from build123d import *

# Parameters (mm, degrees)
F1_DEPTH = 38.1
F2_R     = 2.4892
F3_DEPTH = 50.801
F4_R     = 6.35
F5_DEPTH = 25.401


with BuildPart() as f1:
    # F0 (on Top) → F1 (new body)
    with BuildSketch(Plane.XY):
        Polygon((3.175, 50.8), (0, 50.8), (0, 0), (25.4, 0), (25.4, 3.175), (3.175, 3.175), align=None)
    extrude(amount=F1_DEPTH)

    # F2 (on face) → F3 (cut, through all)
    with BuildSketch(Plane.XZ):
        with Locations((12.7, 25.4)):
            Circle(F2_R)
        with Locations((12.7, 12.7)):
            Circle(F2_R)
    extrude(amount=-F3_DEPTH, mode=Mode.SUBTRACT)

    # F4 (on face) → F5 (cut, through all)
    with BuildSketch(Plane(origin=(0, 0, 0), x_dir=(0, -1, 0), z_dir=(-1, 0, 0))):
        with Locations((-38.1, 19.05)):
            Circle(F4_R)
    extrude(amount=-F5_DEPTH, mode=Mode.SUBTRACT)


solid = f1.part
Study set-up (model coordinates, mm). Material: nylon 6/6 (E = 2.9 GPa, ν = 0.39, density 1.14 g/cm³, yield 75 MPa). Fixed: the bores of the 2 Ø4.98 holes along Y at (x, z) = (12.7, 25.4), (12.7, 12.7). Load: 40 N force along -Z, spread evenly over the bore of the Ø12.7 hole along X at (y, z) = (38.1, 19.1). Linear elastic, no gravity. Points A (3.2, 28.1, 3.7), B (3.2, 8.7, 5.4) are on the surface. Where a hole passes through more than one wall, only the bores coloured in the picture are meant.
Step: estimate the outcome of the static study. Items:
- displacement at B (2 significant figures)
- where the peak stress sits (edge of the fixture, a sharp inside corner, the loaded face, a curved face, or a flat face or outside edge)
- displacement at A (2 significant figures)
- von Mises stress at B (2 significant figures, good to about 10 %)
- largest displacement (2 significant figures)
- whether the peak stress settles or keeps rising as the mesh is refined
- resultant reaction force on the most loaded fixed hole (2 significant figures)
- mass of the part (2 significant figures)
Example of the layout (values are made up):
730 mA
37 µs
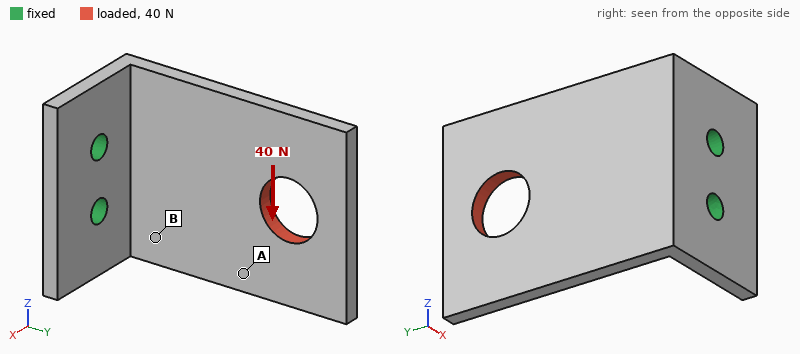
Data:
0.19 mm
edge of the fixture
0.41 mm
4.9 MPa
0.69 mm
keeps rising
81 N
9.5 g
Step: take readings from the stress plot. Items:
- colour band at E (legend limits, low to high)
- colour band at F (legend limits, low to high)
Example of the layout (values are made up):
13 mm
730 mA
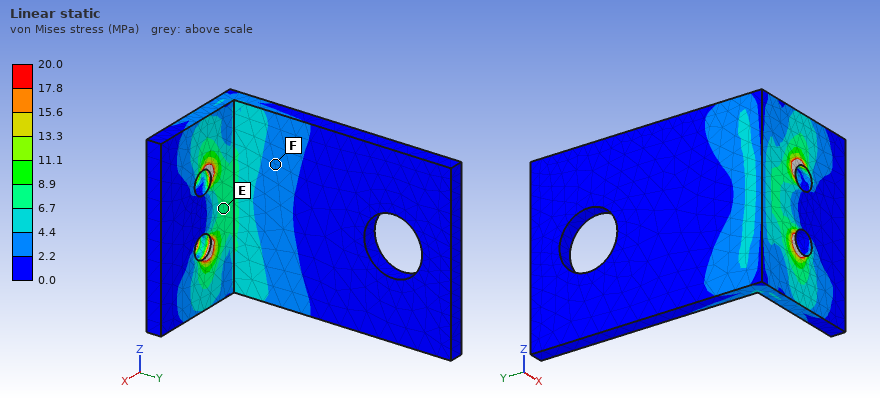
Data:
6.7 to 8.9 MPa
2.2 to 4.4 MPa
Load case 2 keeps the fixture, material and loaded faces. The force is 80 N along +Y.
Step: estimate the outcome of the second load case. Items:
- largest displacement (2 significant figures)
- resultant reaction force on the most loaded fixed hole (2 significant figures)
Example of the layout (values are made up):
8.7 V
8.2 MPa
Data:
0.68 mm
40 N
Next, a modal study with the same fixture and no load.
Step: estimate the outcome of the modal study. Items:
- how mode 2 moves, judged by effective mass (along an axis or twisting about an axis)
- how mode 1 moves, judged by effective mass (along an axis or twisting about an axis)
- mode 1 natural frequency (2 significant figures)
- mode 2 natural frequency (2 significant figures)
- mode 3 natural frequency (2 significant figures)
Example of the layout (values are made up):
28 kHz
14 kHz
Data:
along Z
along X
280 Hz
680 Hz
950 Hz
